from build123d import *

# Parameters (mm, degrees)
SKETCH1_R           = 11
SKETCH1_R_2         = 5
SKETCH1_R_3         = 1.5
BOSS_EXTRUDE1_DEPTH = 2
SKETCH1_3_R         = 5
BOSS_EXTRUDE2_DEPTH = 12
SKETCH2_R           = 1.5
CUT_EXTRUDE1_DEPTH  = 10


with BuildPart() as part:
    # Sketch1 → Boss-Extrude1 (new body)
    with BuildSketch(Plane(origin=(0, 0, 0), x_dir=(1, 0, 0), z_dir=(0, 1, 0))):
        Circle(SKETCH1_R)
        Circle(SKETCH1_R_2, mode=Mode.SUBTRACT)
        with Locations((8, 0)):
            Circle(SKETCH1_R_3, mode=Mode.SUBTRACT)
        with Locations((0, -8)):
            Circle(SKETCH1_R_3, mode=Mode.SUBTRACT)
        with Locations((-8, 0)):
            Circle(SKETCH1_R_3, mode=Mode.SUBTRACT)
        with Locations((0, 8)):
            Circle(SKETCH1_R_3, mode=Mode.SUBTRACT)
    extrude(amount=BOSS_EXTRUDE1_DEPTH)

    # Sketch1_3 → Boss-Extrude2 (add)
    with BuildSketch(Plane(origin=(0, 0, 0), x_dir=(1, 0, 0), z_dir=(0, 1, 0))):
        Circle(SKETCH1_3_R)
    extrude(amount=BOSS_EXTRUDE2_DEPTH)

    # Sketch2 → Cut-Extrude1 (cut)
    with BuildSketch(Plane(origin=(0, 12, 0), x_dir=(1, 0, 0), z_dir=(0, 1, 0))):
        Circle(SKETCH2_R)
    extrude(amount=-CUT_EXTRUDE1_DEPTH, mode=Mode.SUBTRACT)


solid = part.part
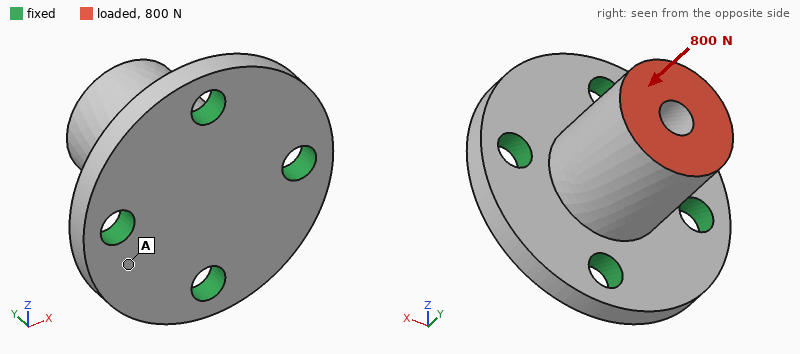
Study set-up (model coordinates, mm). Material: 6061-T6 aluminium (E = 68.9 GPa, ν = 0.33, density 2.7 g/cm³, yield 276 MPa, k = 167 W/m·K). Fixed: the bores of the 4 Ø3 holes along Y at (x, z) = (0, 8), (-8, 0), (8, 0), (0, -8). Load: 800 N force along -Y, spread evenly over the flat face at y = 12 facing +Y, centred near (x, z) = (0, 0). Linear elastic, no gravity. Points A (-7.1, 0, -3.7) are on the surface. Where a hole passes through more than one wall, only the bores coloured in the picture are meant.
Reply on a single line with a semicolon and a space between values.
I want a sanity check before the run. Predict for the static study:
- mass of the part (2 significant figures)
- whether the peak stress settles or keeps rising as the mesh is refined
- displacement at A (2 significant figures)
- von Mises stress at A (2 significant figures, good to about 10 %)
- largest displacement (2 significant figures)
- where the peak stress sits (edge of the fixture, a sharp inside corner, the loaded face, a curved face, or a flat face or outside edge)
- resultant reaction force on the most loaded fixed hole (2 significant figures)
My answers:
3.8 g; keeps rising; 0.96 µm; 13 MPa; 5.0 µm; edge of the fixture; 210 N
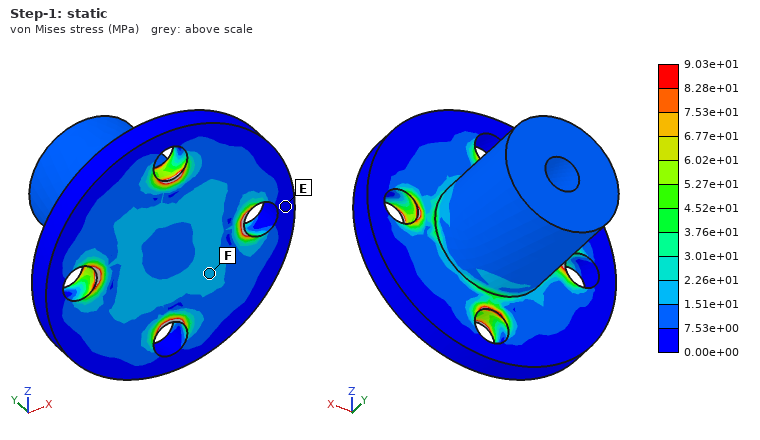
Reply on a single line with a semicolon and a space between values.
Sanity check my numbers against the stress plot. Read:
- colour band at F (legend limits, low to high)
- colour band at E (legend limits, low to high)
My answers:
1.51e+01 to 2.26e+01 MPa; 0.00e+00 to 7.53e+00 MPa
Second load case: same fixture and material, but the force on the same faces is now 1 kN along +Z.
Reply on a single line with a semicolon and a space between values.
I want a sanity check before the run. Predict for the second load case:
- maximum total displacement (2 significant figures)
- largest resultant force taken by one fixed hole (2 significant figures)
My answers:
48 µm; 900 N
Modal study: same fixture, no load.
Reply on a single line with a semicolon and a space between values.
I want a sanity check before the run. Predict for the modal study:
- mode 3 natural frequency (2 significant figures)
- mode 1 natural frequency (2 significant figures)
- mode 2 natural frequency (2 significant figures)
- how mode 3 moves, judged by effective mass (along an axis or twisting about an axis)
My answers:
46 kHz; 28 kHz; 28 kHz; along Y
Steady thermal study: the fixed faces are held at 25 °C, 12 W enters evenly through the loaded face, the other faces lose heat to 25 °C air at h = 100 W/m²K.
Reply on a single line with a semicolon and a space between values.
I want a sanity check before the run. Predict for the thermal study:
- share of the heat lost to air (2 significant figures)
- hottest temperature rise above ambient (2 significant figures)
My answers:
3.9 %; 14 K
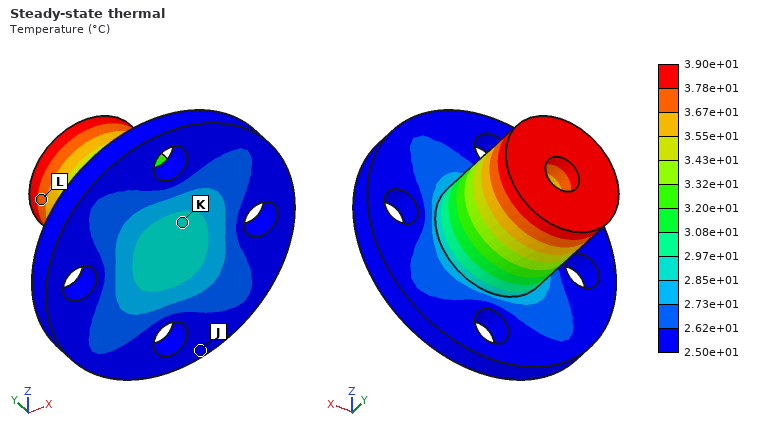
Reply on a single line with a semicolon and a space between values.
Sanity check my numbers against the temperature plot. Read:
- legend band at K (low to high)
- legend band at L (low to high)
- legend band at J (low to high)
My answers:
2.85e+01 to 2.97e+01 °C; 3.67e+01 to 3.78e+01 °C; 2.50e+01 to 2.62e+01 °C
